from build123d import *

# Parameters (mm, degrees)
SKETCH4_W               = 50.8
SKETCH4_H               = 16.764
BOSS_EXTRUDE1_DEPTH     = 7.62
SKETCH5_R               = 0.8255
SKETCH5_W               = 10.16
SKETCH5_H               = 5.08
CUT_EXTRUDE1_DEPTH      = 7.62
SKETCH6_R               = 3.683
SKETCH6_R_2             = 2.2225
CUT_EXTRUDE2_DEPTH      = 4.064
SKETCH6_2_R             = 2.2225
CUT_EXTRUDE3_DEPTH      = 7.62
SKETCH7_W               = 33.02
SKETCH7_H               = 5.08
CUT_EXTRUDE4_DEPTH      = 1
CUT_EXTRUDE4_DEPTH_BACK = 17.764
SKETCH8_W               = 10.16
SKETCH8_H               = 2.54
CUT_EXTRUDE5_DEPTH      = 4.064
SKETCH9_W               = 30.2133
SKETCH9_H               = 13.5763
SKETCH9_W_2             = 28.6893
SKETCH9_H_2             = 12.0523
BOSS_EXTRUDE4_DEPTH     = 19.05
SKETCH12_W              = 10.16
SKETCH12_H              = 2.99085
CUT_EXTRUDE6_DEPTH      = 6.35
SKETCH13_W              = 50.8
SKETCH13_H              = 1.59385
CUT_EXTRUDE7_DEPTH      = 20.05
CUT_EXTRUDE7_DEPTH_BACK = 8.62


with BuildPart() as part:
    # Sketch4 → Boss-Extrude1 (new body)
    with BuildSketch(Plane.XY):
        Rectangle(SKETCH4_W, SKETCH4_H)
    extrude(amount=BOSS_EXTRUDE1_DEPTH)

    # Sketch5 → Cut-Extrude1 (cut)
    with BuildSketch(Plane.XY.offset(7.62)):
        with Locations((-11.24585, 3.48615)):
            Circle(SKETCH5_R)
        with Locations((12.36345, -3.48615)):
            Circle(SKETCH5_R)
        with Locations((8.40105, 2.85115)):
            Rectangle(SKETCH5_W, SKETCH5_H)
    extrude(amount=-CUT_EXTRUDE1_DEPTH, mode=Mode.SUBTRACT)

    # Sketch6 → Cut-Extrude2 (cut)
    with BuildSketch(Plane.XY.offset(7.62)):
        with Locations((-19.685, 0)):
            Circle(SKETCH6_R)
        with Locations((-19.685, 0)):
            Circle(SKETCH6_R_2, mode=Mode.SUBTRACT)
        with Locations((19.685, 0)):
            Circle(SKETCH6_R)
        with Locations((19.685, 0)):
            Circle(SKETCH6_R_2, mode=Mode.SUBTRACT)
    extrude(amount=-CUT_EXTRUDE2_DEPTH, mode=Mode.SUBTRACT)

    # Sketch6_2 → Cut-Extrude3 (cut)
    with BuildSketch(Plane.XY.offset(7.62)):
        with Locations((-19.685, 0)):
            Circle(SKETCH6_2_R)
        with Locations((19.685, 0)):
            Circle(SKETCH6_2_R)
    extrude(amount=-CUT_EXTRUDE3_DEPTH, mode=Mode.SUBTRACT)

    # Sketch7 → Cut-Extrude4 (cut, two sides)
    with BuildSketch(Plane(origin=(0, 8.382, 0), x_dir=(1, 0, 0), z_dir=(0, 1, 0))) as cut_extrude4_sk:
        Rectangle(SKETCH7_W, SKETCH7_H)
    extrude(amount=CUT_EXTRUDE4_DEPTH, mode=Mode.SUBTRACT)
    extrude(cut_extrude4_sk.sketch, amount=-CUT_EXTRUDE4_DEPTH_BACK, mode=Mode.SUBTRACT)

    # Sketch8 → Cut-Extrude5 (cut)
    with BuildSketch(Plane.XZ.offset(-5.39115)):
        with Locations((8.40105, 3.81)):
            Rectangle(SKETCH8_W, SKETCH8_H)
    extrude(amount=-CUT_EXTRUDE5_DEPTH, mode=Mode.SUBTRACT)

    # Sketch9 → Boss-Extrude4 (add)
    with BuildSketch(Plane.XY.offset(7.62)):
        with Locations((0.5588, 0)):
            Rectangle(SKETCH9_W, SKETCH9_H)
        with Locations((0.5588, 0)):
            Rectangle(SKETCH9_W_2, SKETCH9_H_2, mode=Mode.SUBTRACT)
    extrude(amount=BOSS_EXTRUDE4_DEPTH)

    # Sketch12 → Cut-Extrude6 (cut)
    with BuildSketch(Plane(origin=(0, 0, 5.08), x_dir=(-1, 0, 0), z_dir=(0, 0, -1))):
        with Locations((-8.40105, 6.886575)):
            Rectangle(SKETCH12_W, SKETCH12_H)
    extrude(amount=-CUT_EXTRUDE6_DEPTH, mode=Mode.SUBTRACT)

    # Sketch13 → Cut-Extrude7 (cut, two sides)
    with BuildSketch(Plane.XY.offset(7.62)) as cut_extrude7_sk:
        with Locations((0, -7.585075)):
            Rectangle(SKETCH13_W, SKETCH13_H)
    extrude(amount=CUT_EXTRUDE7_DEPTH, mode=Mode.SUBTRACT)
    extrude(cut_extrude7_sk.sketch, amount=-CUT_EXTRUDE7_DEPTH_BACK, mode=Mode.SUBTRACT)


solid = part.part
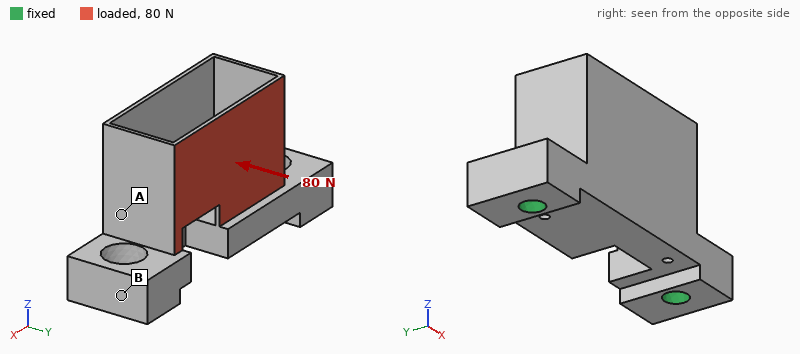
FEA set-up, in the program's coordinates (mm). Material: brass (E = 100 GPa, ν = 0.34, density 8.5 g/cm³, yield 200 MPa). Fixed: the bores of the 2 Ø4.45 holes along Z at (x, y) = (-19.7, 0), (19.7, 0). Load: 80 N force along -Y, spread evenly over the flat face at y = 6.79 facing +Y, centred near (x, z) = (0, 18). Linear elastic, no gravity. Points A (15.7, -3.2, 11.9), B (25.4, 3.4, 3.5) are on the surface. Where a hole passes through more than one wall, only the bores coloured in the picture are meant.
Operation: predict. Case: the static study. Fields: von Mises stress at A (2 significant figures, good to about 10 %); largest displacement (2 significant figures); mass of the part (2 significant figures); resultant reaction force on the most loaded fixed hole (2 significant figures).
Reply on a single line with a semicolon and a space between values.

13 MPa; 0.11 mm; 42 g; 41 N
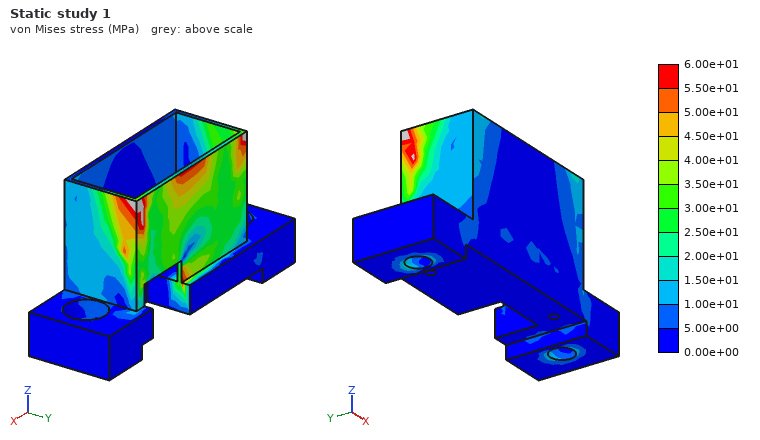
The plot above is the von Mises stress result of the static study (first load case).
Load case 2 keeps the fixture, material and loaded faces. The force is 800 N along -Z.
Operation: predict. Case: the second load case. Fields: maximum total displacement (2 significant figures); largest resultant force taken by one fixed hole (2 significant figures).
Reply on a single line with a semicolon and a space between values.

92 µm; 460 N
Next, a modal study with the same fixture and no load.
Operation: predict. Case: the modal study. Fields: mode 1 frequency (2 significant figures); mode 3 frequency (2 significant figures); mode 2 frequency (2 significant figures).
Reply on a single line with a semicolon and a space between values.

3000 Hz; 6700 Hz; 3300 Hz
